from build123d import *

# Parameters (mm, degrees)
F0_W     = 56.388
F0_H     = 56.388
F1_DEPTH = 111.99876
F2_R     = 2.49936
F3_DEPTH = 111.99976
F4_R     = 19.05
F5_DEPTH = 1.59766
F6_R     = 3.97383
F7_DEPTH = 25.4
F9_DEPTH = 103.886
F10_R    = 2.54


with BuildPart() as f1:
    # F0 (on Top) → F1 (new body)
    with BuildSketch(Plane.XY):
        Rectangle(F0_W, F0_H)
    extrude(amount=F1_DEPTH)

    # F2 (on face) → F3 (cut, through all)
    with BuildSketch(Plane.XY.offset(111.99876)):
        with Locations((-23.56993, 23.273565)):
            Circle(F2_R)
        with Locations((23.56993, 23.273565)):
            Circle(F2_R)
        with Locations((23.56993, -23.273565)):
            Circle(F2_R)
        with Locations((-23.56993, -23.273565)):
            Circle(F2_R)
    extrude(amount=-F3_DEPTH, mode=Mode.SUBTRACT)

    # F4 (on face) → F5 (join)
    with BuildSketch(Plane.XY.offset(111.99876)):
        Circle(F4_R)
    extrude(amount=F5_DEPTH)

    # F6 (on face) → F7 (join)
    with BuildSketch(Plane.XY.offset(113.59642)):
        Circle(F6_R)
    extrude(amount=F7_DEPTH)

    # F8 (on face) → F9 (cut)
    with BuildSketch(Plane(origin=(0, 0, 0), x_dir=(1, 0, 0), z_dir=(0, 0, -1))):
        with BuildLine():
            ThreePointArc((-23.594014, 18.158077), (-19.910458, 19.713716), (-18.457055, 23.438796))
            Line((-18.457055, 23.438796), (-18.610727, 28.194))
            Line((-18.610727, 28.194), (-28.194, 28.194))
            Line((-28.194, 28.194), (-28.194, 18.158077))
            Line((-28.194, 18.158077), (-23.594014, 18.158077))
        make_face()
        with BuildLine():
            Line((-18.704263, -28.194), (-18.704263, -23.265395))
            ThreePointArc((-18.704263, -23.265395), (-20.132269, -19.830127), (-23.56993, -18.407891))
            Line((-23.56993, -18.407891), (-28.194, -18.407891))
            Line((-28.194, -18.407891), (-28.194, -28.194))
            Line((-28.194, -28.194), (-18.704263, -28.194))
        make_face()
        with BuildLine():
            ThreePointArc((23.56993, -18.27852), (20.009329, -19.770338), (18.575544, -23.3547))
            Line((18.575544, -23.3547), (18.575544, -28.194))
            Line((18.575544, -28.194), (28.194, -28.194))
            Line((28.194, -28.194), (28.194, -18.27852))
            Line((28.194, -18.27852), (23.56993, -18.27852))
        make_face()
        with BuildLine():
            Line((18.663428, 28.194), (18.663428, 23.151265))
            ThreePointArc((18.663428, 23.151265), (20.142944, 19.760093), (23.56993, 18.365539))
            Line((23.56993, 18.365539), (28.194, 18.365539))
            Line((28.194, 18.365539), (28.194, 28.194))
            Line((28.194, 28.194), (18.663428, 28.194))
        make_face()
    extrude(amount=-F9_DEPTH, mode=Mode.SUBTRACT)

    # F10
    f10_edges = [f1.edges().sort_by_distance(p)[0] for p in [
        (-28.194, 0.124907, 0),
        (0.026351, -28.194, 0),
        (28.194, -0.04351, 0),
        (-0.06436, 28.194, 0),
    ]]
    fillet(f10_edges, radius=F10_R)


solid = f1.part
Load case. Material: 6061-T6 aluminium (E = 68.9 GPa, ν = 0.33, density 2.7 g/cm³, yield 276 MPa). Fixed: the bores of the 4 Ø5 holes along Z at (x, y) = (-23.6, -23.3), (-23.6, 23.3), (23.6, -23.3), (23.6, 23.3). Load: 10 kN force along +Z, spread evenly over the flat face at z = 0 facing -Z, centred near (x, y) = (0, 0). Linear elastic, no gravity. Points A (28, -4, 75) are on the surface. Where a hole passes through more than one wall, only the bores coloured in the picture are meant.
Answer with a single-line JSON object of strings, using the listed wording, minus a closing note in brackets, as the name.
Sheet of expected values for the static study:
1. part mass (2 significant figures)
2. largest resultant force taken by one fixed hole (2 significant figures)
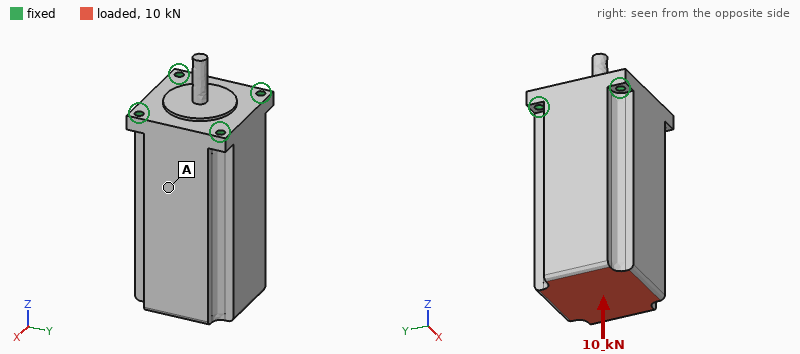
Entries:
{"part mass": "870 g", "largest resultant force taken by one fixed hole": "2.7 kN"}
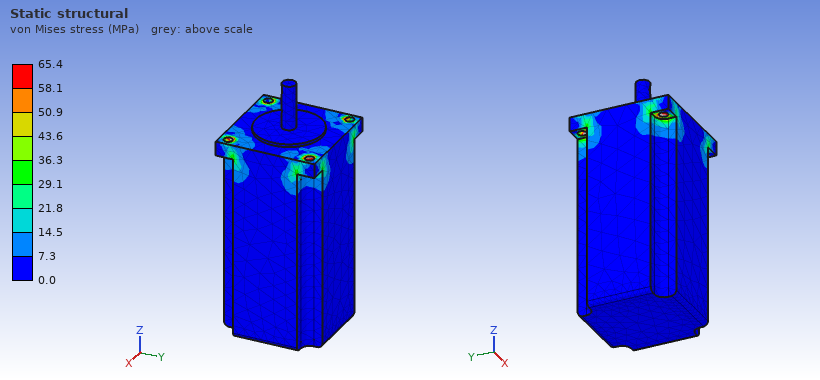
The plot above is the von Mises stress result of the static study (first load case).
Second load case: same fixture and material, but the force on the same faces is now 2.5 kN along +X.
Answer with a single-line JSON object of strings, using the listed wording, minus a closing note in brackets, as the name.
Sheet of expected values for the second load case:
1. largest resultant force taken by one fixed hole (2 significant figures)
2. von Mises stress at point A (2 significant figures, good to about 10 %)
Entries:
{"largest resultant force taken by one fixed hole": "3.2 kN", "von Mises stress at point A": "7.8 MPa"}
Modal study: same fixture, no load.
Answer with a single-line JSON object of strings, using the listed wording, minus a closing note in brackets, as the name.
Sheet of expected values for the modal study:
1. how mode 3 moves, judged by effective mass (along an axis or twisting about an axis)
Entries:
{"how mode 3 moves, judged by effective mass": "along Z"}
